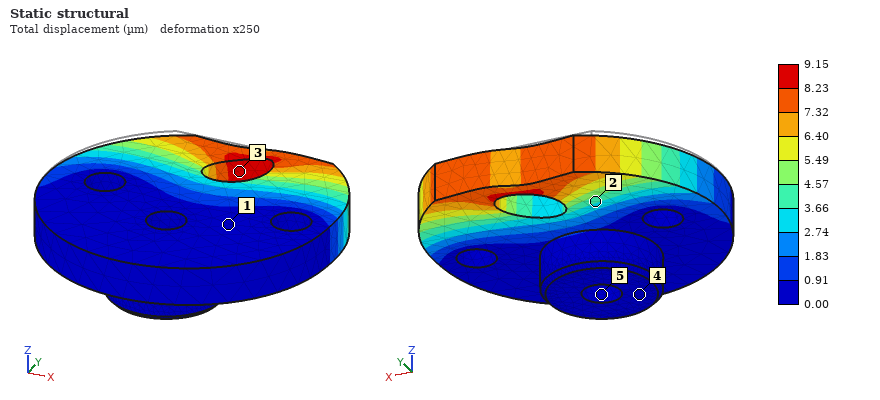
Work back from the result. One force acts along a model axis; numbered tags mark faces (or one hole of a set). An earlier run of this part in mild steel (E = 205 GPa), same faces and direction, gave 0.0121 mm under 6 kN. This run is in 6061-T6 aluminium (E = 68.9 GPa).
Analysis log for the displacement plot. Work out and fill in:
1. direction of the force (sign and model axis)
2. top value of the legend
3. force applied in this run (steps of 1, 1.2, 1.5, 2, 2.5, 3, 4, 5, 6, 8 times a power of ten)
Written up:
+X
9.15 µm
1.5 kN
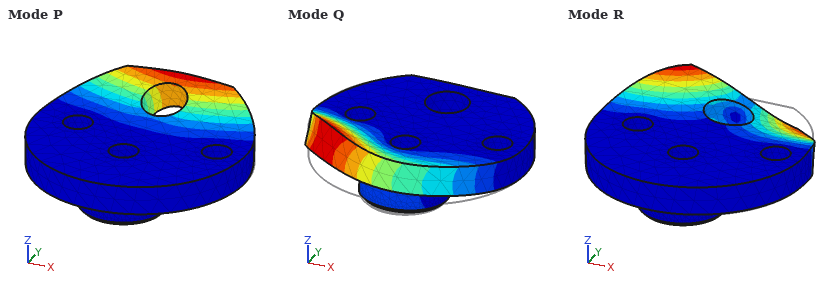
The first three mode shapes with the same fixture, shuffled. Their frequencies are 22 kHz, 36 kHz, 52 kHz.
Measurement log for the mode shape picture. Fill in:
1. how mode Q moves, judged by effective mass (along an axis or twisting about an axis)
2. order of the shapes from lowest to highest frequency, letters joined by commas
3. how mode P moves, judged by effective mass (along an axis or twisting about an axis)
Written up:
along Z
P, R, Q
along Z
